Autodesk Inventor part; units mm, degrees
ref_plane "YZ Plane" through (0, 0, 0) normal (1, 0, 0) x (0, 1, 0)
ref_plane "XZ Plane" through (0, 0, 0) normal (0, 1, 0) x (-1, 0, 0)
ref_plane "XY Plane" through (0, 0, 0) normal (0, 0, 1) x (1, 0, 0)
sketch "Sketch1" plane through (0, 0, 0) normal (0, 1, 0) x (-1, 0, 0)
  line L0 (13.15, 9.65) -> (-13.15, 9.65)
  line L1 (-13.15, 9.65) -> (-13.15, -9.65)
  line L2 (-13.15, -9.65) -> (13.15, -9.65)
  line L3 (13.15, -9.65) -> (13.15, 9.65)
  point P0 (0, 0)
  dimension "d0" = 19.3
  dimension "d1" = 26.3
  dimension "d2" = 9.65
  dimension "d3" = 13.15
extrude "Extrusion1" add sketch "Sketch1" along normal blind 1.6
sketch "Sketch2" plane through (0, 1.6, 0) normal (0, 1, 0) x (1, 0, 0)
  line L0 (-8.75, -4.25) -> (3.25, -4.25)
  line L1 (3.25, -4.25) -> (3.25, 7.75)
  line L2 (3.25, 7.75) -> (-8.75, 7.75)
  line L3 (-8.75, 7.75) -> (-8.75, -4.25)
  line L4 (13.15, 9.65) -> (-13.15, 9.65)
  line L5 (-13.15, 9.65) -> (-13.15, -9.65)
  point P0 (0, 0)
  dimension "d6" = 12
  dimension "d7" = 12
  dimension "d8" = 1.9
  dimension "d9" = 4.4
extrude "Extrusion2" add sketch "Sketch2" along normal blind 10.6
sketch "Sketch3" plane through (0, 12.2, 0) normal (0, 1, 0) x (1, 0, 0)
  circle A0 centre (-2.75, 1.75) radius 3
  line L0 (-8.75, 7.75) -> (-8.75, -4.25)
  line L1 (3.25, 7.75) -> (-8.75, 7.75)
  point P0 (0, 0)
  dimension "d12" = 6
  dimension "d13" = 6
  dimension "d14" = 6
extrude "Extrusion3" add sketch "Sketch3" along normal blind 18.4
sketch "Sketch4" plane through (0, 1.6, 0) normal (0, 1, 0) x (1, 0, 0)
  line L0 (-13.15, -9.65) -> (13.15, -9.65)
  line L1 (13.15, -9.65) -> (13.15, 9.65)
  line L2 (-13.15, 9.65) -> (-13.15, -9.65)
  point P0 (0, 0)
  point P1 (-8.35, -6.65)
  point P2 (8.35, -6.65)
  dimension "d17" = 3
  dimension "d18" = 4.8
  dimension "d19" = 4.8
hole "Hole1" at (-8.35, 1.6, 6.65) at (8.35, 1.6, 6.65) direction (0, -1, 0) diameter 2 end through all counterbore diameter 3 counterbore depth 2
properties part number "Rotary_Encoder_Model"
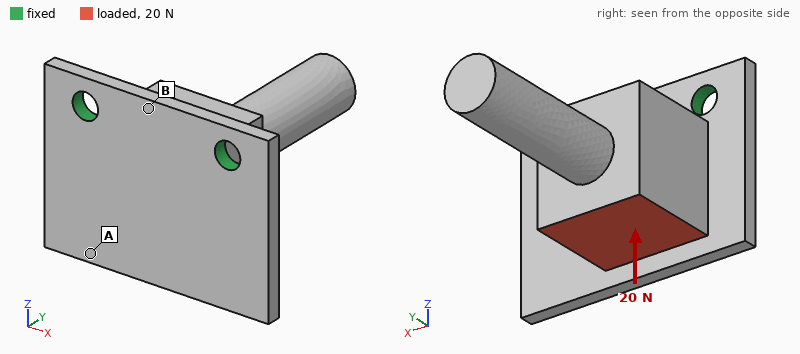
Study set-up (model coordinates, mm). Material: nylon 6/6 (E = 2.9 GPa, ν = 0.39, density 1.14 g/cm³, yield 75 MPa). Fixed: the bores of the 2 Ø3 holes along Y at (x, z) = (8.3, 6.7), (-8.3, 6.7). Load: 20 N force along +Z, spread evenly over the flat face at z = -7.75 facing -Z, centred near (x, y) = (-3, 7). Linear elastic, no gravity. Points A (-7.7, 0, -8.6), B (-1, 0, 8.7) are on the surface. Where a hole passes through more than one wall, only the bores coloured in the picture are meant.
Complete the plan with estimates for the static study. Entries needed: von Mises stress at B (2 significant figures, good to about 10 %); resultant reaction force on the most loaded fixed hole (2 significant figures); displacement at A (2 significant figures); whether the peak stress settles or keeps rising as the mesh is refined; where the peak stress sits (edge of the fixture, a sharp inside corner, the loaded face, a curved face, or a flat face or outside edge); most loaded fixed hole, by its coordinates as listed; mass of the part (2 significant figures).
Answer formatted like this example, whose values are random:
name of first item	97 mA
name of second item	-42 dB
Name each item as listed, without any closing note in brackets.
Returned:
von Mises stress at B	4.2 MPa
resultant reaction force on the most loaded fixed hole	14 N
displacement at A	0.22 mm
whether the peak stress settles or keeps rising as the mesh is refined	keeps rising
where the peak stress sits	edge of the fixture
most loaded fixed hole, by its coordinates as listed	(-8.3, 6.7)
mass of the part	3.2 g
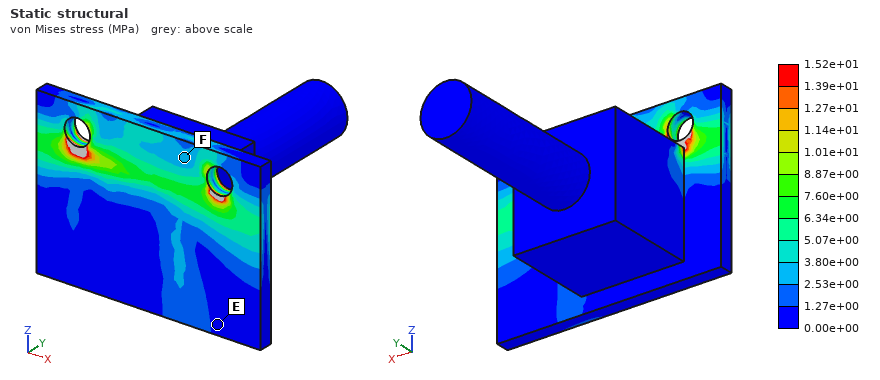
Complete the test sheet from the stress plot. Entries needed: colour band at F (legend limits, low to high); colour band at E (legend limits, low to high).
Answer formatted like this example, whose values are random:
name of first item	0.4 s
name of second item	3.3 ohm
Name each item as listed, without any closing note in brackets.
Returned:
colour band at F	2.53e+00 to 3.80e+00 MPa
colour band at E	0.00e+00 to 1.27e+00 MPa
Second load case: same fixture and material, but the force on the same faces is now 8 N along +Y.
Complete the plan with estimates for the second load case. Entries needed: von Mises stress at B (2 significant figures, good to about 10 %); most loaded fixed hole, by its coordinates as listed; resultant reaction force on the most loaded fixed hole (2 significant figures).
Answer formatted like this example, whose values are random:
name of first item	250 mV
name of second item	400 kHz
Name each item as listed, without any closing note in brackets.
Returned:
von Mises stress at B	2.8 MPa
most loaded fixed hole, by its coordinates as listed	(-8.3, 6.7)
resultant reaction force on the most loaded fixed hole	4.6 N
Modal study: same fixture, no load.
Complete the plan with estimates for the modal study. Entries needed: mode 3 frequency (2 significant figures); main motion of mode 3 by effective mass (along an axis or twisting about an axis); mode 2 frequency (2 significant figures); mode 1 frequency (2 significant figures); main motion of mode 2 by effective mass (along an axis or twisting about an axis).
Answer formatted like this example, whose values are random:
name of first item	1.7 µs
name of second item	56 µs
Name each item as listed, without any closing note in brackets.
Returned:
mode 3 frequency	3700 Hz
main motion of mode 3 by effective mass	along Y
mode 2 frequency	1700 Hz
mode 1 frequency	590 Hz
main motion of mode 2 by effective mass	along X
